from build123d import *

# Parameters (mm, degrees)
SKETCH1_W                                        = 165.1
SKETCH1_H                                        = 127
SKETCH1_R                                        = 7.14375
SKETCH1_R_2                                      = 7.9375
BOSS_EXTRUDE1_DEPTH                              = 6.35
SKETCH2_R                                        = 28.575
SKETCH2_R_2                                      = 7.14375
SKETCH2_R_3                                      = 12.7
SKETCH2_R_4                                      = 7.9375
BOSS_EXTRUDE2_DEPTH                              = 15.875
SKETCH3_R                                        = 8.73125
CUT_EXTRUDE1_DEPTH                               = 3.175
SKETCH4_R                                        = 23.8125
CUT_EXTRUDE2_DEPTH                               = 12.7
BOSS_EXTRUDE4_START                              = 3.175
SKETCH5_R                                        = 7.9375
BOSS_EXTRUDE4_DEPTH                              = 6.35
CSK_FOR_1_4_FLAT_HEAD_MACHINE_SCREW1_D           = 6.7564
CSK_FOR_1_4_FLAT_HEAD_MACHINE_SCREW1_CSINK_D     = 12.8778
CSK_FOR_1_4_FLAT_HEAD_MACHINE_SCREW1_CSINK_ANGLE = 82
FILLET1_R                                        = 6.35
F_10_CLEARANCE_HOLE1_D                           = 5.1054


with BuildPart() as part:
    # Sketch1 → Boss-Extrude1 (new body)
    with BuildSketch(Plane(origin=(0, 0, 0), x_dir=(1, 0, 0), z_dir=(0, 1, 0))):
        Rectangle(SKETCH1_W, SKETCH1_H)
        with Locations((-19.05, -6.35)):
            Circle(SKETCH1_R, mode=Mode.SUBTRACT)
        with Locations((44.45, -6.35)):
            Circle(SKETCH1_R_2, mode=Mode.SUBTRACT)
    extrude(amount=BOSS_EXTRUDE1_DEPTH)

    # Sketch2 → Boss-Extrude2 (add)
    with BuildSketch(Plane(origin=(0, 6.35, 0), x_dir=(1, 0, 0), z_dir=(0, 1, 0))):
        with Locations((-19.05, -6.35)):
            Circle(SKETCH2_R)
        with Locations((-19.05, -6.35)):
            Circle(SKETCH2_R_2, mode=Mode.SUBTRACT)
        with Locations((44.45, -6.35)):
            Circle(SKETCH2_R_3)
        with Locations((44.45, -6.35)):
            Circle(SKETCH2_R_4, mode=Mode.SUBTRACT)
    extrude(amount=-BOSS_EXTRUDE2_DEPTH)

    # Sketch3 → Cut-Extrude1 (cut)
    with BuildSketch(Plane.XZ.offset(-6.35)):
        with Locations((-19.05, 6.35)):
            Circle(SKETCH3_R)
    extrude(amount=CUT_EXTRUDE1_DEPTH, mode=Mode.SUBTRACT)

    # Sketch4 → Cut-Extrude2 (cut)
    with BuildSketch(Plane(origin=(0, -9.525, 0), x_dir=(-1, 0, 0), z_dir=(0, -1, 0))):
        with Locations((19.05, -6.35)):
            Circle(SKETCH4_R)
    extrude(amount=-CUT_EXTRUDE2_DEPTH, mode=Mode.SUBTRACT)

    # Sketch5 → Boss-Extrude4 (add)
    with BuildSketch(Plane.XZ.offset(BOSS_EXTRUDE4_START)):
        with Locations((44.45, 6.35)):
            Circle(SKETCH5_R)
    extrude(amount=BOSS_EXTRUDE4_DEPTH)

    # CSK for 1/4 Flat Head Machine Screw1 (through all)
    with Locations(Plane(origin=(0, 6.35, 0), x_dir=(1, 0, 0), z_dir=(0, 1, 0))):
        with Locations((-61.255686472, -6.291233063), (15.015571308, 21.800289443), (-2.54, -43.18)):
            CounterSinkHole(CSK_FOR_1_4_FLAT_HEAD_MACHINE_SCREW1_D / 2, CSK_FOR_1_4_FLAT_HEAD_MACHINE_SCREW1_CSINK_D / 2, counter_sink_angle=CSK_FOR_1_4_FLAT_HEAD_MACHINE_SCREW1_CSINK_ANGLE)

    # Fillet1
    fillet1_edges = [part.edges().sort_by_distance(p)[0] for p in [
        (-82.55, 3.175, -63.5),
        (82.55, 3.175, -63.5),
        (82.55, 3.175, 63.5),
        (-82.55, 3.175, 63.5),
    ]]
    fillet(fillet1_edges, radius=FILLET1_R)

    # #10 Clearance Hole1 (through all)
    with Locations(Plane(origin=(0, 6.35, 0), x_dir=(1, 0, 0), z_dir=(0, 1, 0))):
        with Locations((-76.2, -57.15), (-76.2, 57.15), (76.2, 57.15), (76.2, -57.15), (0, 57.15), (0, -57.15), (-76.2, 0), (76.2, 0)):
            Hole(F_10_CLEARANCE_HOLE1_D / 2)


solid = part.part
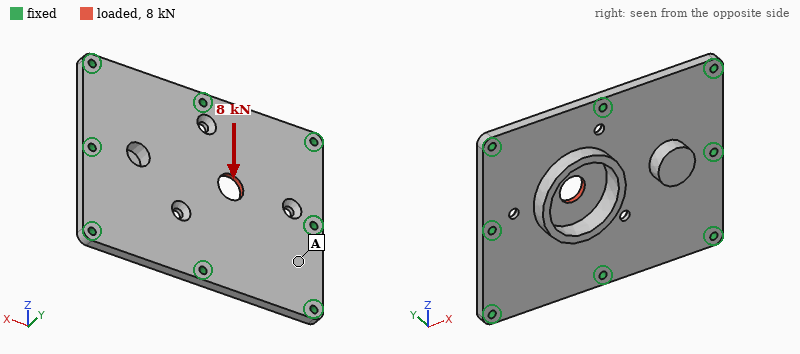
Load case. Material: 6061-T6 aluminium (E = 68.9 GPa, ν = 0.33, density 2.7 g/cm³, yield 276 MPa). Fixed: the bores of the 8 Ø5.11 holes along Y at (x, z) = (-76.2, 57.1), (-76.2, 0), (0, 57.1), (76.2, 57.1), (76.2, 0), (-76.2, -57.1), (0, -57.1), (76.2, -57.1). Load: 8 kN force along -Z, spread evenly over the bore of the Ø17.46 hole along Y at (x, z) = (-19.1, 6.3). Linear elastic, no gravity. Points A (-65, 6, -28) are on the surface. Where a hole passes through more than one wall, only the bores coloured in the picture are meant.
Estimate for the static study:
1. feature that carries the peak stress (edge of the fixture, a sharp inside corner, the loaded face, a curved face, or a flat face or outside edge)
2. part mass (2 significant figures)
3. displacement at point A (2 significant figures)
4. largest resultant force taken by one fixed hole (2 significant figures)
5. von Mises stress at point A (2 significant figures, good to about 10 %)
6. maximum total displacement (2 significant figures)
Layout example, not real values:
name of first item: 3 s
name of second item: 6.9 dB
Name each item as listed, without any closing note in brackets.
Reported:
feature that carries the peak stress: the loaded face
part mass: 360 g
displacement at point A: 3.3 µm
largest resultant force taken by one fixed hole: 2.2 kN
von Mises stress at point A: 6.9 MPa
maximum total displacement: 20 µm
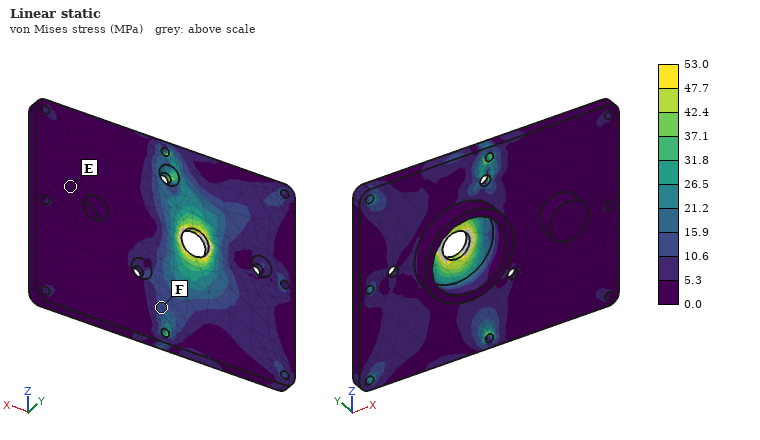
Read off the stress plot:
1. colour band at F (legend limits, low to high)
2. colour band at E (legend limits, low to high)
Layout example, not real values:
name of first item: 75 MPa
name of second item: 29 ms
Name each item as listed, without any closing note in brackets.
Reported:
colour band at F: 10.6 to 15.9 MPa
colour band at E: 0.0 to 5.3 MPa
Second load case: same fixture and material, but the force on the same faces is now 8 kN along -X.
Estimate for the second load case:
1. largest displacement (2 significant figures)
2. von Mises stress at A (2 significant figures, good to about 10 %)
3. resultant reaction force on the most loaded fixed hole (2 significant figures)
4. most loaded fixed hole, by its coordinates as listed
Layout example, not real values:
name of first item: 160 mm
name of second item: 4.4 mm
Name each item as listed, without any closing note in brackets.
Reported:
largest displacement: 19 µm
von Mises stress at A: 4.7 MPa
resultant reaction force on the most loaded fixed hole: 1.9 kN
most loaded fixed hole, by its coordinates as listed: (-76.2, 0)
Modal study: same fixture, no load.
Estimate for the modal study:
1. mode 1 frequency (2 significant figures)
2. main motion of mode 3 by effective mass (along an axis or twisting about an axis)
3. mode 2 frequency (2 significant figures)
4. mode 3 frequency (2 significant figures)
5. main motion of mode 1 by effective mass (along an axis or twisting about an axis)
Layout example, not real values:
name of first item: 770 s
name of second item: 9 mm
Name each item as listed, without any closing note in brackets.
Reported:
mode 1 frequency: 2700 Hz
main motion of mode 3 by effective mass: twisting about X
mode 2 frequency: 4000 Hz
mode 3 frequency: 4800 Hz
main motion of mode 1 by effective mass: along Y
